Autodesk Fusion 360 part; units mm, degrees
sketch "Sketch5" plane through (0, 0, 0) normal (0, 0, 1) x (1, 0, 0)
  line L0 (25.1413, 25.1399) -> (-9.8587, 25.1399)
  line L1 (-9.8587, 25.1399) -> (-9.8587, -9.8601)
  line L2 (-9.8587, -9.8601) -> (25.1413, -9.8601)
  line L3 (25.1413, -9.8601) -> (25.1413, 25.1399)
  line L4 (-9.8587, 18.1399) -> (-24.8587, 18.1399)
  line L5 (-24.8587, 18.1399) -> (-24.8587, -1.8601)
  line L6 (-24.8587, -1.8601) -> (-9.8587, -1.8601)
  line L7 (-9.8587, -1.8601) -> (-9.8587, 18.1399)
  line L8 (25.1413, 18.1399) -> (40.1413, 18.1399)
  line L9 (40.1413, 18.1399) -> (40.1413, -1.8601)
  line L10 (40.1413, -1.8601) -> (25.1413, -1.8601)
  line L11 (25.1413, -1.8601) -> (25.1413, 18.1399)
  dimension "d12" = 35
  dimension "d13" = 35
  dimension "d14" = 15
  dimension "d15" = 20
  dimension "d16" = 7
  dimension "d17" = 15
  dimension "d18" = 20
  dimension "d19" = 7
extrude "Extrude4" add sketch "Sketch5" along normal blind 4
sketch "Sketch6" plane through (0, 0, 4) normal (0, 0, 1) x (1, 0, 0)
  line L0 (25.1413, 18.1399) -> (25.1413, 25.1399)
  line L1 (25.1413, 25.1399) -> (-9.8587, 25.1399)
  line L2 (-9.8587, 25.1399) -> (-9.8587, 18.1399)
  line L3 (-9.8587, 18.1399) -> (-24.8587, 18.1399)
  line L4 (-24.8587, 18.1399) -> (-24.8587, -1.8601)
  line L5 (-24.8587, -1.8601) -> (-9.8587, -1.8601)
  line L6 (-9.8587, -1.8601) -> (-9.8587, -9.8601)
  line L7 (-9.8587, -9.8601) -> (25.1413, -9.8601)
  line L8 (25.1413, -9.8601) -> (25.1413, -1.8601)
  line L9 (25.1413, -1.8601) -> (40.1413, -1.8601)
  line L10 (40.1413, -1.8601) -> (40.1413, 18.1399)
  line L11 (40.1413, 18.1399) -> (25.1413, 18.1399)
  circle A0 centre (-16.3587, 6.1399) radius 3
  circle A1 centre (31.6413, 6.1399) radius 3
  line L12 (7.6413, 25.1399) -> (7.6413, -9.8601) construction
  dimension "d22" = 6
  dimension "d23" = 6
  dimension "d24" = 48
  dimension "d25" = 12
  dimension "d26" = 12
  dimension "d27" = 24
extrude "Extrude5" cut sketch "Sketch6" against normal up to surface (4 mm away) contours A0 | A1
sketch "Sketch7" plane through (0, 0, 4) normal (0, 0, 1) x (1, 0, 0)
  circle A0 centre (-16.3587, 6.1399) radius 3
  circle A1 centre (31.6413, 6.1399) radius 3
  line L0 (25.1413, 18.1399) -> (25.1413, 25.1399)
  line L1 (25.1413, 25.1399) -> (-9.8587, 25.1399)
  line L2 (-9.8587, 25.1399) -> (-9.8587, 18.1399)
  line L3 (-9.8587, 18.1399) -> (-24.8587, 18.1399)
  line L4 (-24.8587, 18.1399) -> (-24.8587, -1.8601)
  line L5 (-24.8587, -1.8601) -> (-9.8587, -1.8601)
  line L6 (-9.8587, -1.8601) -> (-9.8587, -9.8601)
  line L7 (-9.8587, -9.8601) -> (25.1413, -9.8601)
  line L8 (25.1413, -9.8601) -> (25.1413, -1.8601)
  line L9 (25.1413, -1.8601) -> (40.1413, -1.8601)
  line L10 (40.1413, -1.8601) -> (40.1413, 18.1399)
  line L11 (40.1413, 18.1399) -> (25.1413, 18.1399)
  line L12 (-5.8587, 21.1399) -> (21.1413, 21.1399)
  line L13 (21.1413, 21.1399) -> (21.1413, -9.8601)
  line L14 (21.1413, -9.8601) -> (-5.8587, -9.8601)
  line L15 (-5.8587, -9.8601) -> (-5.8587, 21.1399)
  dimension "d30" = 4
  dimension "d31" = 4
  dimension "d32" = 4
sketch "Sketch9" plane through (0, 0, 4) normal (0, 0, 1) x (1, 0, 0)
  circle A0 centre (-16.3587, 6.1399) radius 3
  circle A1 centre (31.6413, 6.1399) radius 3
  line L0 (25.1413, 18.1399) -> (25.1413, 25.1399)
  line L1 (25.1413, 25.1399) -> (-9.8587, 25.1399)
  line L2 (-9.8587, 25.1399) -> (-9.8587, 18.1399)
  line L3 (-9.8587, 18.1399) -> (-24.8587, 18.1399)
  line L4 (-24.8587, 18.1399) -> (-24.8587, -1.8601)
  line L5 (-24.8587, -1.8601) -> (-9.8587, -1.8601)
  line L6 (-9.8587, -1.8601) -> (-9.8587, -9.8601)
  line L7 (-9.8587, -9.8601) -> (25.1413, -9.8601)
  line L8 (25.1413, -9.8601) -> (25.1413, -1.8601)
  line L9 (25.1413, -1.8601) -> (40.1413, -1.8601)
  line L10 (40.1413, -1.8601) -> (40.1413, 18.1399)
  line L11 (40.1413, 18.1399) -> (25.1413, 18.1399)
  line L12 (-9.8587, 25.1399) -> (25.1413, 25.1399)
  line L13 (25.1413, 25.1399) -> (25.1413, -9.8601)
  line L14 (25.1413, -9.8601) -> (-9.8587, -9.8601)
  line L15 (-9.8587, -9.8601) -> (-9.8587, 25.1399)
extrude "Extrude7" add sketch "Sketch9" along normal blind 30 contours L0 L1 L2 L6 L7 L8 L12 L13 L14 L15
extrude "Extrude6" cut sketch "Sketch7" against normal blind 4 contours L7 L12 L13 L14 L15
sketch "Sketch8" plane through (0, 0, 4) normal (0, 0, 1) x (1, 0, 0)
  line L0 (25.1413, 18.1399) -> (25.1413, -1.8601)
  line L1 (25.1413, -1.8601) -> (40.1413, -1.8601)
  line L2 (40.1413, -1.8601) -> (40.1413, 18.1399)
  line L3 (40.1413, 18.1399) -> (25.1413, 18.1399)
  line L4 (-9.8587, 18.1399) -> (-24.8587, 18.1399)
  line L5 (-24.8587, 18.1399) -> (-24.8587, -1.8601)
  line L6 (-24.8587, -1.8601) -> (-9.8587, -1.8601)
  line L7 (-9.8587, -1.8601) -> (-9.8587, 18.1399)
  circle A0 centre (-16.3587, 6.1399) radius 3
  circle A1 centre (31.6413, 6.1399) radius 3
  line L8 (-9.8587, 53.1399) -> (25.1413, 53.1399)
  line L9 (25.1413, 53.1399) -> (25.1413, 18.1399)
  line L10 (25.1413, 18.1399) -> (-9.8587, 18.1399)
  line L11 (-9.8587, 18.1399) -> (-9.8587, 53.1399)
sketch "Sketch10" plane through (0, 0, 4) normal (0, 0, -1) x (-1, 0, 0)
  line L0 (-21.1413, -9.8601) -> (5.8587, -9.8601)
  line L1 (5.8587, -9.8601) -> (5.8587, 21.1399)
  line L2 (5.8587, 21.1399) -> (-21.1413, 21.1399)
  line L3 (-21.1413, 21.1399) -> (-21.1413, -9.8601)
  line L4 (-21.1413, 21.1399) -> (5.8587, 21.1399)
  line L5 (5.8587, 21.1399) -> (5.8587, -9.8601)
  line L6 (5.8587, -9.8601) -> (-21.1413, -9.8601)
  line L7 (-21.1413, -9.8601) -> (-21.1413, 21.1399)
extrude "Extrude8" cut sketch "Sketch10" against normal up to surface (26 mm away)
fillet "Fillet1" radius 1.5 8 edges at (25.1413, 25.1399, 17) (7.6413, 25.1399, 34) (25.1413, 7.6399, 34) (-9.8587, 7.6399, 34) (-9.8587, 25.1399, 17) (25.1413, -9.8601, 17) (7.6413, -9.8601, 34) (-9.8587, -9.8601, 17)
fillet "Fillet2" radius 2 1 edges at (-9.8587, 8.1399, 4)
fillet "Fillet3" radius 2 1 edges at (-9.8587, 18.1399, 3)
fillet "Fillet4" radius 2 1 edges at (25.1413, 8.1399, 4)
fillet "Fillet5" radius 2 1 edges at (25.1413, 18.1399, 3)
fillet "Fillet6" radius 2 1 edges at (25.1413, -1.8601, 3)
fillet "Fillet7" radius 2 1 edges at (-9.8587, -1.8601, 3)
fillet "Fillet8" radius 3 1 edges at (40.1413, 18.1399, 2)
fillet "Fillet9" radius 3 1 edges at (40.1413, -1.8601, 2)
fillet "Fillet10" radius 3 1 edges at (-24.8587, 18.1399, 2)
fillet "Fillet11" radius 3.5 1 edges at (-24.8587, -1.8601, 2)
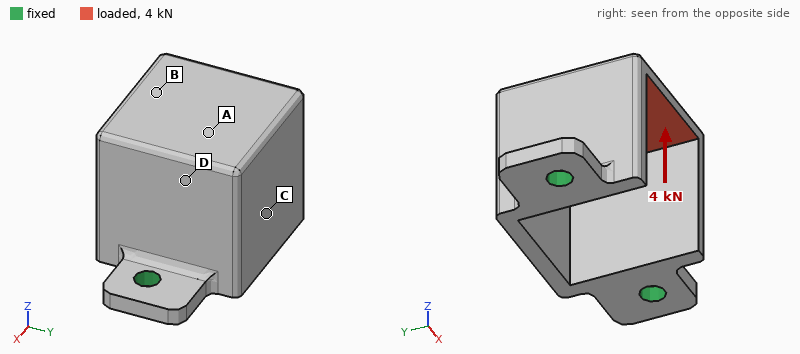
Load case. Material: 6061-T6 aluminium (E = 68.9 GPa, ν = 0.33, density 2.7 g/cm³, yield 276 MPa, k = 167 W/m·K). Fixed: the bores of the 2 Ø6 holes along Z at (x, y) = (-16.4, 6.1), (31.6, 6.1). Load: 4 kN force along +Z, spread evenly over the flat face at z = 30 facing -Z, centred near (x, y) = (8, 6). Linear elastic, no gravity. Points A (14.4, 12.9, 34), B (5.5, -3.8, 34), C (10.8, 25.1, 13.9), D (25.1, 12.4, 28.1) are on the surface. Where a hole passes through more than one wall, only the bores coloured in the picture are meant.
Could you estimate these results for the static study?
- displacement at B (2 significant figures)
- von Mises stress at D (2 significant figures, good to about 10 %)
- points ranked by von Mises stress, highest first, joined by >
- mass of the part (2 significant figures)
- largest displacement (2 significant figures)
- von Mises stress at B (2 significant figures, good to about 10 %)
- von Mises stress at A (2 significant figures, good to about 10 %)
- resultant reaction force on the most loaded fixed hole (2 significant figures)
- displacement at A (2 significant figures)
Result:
0.090 mm
32 MPa
B > A > D > C
50 g
0.11 mm
88 MPa
46 MPa
2.1 kN
0.049 mm
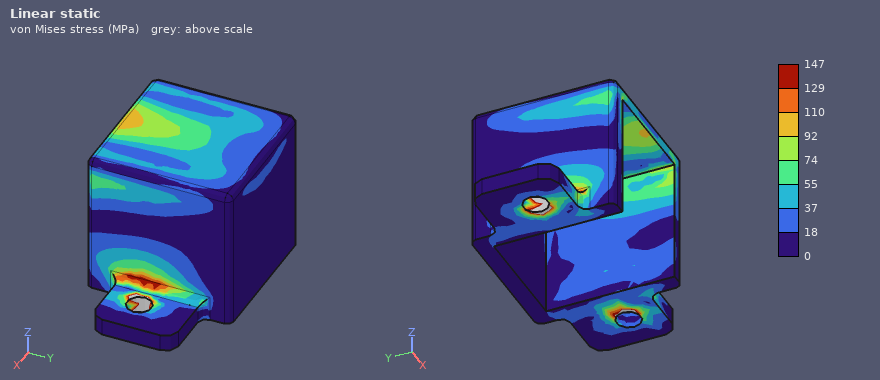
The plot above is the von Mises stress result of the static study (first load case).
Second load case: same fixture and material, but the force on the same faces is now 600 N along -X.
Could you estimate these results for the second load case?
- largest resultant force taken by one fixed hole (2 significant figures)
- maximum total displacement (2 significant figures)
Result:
460 N
91 µm
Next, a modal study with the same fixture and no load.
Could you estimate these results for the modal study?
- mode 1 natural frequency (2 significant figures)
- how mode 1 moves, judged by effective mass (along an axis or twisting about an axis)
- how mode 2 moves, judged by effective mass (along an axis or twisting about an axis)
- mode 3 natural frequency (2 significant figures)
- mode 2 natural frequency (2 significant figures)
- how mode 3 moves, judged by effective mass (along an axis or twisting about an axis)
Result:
2200 Hz
along Y
along X
8200 Hz
3300 Hz
along X
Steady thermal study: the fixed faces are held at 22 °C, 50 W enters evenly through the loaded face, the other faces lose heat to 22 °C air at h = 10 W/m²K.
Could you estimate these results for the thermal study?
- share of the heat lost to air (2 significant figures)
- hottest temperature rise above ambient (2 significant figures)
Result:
4.7 %
49 K
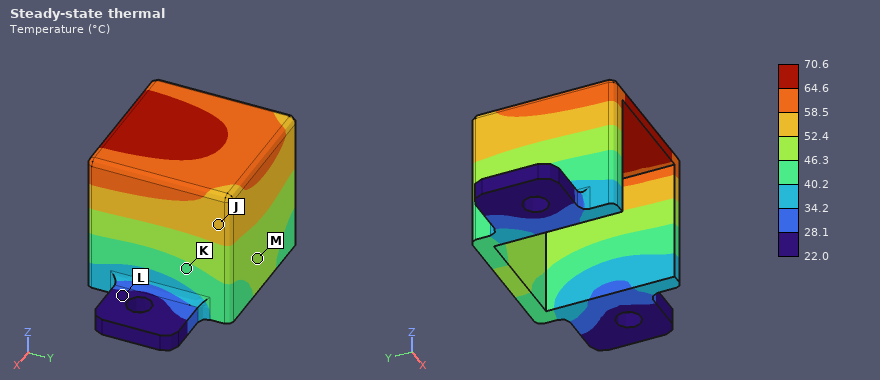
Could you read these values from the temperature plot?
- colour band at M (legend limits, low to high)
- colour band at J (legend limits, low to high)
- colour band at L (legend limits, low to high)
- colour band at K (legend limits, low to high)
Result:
46.3 to 52.4 °C
52.4 to 58.5 °C
22.0 to 28.1 °C
40.2 to 46.3 °C
